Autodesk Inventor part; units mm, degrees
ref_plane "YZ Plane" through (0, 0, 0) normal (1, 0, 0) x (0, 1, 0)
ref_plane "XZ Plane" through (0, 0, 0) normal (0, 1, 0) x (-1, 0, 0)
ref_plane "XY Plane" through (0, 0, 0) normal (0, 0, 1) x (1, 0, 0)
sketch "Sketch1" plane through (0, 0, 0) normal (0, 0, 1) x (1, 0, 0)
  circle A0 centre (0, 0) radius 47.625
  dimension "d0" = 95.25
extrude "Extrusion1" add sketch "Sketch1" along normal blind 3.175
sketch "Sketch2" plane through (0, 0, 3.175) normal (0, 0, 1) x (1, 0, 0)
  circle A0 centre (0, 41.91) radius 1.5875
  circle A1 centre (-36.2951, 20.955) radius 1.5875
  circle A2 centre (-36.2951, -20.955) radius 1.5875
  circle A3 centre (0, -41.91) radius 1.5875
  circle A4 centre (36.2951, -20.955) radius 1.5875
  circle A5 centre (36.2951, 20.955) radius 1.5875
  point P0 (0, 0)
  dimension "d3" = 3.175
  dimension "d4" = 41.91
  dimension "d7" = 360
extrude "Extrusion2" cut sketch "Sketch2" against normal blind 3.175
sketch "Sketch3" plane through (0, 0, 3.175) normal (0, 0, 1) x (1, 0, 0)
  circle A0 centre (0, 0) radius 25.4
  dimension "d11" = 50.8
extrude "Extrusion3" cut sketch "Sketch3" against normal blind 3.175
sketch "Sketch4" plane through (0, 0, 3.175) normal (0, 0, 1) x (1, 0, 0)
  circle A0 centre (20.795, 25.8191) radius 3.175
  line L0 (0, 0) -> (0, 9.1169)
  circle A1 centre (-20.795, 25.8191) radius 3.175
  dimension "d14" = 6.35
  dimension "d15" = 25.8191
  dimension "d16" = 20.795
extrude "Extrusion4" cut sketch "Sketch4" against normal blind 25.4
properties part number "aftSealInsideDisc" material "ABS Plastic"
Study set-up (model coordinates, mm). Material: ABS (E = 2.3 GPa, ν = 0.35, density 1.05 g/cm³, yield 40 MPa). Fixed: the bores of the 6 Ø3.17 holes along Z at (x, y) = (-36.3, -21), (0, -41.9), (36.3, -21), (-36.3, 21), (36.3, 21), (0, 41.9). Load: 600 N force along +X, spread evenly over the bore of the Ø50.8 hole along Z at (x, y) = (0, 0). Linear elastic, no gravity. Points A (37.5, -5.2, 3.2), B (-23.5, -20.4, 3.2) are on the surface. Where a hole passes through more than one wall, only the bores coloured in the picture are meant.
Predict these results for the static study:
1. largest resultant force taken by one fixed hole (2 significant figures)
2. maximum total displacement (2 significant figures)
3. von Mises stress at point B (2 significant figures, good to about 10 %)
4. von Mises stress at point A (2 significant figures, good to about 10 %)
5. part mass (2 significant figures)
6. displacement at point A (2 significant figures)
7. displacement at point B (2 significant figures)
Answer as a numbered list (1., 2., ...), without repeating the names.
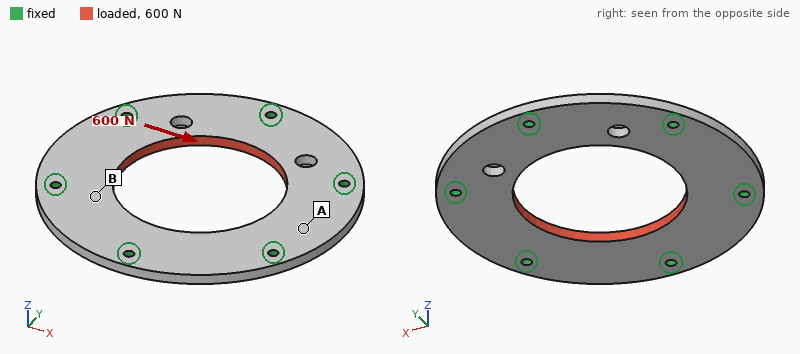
1. 120 N
2. 27 µm
3. 2.1 MPa
4. 0.72 MPa
5. 17 g
6. 21 µm
7. 13 µm
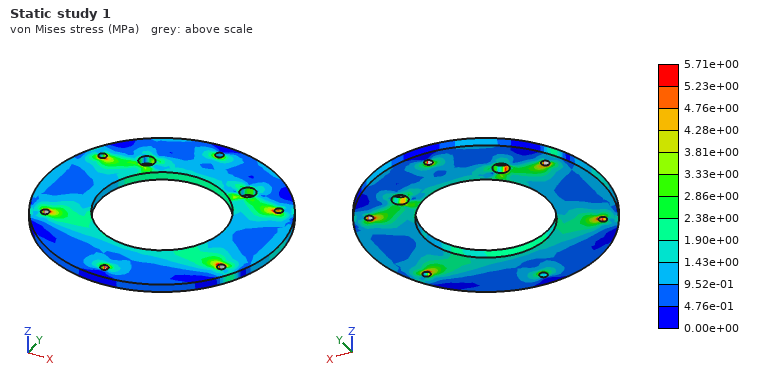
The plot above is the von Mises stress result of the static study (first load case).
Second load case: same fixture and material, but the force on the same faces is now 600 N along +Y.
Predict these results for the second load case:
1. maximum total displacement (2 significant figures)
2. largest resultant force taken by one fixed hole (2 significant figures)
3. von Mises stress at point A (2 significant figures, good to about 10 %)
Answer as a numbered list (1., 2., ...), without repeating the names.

1. 27 µm
2. 130 N
3. 0.82 MPa
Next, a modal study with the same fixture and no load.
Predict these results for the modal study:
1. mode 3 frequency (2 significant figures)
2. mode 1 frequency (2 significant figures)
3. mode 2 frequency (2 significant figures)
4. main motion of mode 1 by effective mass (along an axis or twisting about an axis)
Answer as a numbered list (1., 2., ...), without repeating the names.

1. 2400 Hz
2. 2100 Hz
3. 2300 Hz
4. along Z
